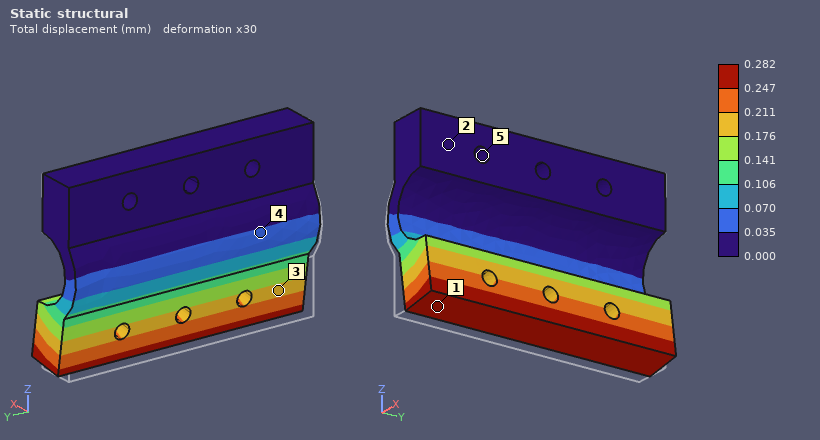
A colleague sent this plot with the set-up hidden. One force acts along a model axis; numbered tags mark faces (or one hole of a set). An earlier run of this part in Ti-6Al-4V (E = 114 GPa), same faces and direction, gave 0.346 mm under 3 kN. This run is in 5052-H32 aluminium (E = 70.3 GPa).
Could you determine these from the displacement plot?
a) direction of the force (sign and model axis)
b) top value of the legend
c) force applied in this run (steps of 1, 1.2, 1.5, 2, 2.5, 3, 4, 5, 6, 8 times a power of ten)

+X
0.282 mm
1.5 kN
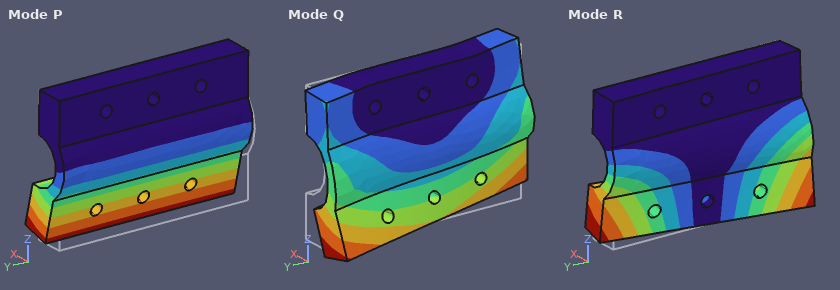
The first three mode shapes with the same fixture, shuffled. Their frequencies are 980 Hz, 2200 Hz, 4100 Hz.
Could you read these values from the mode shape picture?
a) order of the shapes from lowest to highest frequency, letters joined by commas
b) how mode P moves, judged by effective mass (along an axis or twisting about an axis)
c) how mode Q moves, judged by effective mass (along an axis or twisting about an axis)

P, R, Q
along X
along Y
